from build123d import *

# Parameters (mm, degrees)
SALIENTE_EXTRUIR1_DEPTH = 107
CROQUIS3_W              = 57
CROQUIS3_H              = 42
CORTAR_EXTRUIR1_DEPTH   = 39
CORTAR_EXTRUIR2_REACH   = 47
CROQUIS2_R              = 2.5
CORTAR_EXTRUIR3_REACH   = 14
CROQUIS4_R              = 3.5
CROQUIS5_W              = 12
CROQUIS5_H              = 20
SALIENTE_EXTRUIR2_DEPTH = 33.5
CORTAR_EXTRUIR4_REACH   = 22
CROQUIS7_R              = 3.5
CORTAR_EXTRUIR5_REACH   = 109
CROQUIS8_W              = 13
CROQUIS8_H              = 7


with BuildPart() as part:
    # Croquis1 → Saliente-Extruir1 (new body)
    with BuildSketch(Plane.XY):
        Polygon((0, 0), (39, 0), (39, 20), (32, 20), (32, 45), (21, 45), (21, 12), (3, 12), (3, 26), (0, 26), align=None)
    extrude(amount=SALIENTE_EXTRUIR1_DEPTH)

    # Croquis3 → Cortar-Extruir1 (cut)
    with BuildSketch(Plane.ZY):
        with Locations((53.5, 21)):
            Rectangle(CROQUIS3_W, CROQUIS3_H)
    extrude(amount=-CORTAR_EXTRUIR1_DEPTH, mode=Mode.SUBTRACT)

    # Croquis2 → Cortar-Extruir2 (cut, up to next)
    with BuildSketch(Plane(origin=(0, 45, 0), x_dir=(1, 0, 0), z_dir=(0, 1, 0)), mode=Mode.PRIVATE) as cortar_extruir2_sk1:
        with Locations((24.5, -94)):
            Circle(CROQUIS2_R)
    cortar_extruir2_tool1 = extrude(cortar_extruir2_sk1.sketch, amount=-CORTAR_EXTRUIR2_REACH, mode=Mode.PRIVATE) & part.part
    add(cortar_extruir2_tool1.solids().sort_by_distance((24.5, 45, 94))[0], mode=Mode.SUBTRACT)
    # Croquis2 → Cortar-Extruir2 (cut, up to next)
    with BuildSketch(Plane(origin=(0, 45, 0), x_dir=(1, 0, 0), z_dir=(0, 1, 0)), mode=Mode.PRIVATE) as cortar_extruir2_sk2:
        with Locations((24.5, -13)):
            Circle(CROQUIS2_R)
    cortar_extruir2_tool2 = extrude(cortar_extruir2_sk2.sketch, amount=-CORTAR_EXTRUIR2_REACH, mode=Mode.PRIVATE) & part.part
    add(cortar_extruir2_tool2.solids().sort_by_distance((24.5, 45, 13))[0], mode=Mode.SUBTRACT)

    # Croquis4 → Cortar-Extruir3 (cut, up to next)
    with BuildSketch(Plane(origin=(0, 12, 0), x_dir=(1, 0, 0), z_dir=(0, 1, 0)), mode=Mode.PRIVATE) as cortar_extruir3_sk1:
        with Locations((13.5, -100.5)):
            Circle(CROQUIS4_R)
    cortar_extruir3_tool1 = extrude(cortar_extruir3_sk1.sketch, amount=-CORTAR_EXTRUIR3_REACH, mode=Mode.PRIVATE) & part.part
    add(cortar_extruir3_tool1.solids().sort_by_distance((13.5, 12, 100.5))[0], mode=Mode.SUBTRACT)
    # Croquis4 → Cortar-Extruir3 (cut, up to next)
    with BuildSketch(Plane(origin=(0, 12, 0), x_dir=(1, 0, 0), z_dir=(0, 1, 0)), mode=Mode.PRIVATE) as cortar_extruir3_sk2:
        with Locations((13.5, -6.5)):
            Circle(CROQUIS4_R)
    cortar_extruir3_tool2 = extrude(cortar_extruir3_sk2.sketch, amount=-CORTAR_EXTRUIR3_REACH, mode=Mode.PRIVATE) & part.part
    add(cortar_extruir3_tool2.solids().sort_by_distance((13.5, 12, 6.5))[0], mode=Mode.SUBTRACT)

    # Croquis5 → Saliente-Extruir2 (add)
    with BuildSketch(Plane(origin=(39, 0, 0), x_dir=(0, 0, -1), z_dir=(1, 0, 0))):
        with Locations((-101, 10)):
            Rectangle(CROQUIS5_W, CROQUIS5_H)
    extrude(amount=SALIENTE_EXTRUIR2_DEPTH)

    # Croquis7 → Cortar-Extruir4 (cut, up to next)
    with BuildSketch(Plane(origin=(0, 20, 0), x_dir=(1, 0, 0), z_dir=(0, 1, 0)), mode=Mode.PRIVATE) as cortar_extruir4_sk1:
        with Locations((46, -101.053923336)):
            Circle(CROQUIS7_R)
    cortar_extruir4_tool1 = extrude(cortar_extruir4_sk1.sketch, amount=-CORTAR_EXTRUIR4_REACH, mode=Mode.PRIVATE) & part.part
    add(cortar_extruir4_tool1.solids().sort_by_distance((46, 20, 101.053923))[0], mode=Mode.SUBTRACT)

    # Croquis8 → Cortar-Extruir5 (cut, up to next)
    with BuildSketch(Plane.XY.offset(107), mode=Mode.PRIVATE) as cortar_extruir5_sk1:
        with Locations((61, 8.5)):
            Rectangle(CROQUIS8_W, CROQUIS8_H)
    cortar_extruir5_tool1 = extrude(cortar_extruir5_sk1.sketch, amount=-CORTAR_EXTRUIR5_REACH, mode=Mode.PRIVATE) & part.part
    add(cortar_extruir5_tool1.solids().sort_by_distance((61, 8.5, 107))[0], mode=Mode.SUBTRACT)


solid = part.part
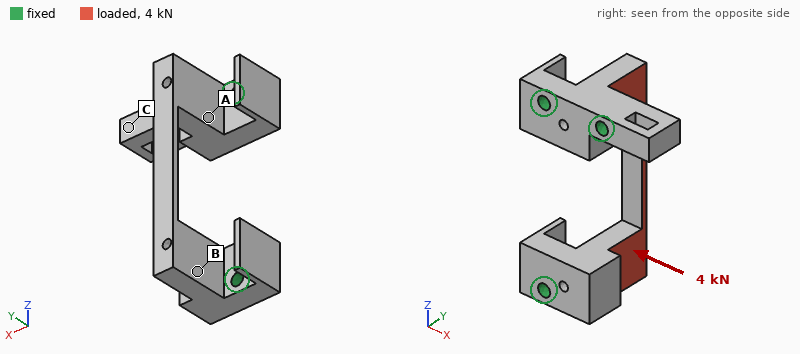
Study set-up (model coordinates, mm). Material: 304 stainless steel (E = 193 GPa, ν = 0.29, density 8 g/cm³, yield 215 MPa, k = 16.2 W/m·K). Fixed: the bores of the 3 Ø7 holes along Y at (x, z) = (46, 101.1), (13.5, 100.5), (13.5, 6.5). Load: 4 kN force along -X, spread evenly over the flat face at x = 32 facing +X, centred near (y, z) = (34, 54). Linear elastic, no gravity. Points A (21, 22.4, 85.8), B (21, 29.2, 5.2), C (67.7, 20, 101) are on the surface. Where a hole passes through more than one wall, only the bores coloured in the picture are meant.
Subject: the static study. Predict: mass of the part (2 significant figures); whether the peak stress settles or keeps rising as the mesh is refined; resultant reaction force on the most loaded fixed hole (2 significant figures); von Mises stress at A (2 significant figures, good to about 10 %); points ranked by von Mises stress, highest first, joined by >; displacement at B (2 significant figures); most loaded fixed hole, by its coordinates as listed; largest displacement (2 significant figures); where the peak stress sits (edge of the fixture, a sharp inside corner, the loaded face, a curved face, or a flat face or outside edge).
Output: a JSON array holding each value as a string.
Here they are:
["410 g", "keeps rising", "2.5 kN", "52 MPa", "A > B > C", "33 µm", "(46, 101.1)", "71 µm", "edge of the fixture"]
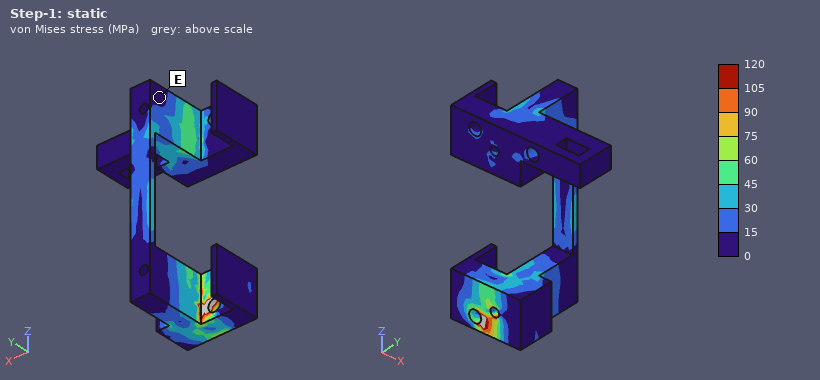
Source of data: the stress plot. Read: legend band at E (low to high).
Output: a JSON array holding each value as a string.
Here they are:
["0 to 15 MPa"]
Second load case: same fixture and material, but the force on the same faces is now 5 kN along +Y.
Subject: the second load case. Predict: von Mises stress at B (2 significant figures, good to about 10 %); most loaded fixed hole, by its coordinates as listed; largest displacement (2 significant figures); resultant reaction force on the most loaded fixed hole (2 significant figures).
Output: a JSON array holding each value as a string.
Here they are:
["11 MPa", "(13.5, 6.5)", "0.11 mm", "2.5 kN"]
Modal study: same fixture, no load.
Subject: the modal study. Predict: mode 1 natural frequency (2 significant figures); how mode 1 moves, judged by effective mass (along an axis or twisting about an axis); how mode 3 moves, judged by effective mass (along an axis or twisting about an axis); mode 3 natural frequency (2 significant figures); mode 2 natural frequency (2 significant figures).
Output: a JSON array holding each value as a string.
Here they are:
["3900 Hz", "along X", "along Z", "5300 Hz", "4200 Hz"]
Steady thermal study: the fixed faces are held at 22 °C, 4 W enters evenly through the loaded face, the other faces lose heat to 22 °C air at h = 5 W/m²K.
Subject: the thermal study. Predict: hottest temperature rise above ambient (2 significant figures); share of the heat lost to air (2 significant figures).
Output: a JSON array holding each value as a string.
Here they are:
["19 K", "11 %"]
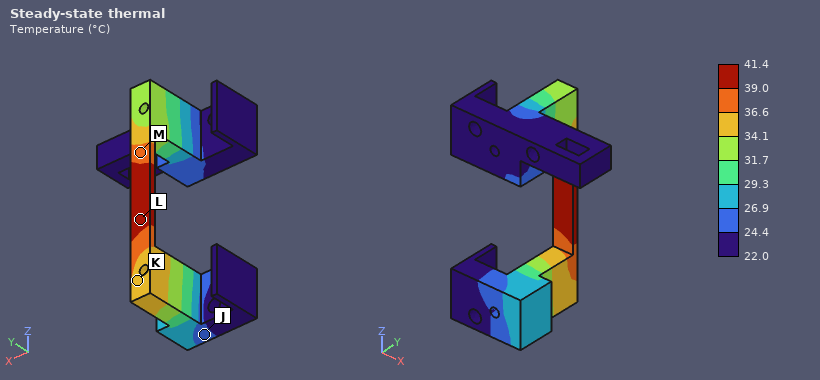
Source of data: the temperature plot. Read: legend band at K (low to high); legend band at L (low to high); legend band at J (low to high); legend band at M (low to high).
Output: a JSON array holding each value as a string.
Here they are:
["34.1 to 36.6 °C", "39.0 to 41.4 °C", "24.4 to 26.9 °C", "36.6 to 39.0 °C"]
